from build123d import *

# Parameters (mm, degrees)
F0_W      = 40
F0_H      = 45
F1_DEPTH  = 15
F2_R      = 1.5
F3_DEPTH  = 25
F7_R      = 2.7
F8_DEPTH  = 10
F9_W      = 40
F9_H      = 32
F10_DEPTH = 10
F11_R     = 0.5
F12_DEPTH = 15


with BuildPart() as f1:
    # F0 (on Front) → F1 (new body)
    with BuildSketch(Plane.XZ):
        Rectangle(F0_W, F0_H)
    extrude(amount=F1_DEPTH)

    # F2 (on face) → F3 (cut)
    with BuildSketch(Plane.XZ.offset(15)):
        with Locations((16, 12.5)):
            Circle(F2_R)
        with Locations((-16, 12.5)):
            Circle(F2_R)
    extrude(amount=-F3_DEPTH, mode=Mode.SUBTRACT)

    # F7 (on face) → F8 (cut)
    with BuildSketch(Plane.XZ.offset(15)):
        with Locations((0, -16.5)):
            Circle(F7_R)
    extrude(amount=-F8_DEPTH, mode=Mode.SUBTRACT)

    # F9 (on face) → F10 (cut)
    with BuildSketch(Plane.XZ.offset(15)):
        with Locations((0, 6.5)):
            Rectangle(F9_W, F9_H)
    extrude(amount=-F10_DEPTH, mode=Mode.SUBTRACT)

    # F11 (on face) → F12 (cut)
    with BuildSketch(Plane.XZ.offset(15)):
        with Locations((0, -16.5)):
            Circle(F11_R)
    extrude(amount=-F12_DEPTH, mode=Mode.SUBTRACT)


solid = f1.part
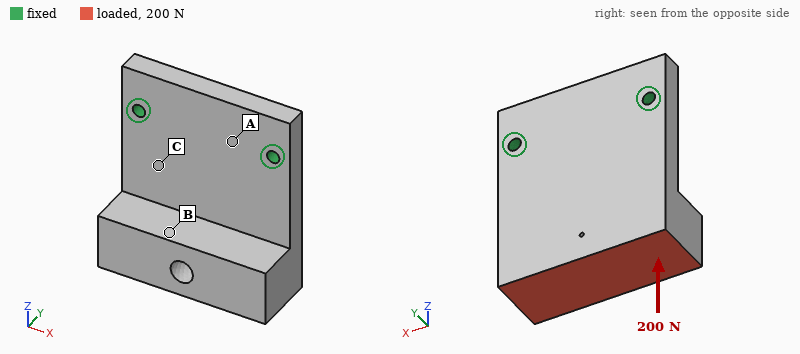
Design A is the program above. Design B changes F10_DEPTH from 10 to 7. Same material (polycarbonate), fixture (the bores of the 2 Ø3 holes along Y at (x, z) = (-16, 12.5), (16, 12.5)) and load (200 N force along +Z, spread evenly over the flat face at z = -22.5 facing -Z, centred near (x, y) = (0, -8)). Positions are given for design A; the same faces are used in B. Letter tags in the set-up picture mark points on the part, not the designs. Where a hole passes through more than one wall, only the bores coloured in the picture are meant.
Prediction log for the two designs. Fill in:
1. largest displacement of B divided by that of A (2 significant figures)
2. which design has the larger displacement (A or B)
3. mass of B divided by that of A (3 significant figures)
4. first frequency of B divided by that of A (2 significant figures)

0.19
A
1.27
1.9
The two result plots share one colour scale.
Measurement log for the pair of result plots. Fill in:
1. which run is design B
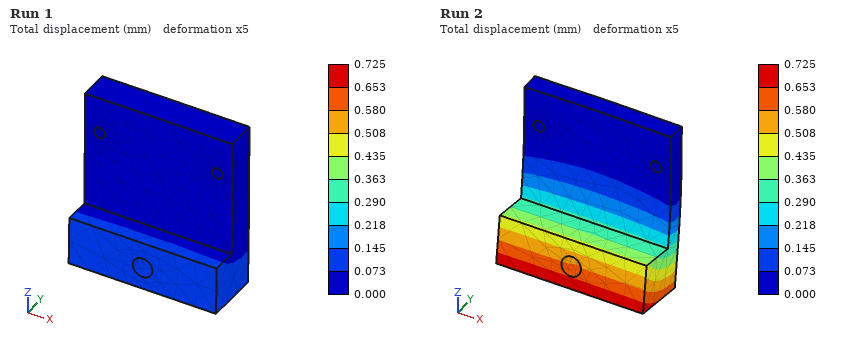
Run 1
